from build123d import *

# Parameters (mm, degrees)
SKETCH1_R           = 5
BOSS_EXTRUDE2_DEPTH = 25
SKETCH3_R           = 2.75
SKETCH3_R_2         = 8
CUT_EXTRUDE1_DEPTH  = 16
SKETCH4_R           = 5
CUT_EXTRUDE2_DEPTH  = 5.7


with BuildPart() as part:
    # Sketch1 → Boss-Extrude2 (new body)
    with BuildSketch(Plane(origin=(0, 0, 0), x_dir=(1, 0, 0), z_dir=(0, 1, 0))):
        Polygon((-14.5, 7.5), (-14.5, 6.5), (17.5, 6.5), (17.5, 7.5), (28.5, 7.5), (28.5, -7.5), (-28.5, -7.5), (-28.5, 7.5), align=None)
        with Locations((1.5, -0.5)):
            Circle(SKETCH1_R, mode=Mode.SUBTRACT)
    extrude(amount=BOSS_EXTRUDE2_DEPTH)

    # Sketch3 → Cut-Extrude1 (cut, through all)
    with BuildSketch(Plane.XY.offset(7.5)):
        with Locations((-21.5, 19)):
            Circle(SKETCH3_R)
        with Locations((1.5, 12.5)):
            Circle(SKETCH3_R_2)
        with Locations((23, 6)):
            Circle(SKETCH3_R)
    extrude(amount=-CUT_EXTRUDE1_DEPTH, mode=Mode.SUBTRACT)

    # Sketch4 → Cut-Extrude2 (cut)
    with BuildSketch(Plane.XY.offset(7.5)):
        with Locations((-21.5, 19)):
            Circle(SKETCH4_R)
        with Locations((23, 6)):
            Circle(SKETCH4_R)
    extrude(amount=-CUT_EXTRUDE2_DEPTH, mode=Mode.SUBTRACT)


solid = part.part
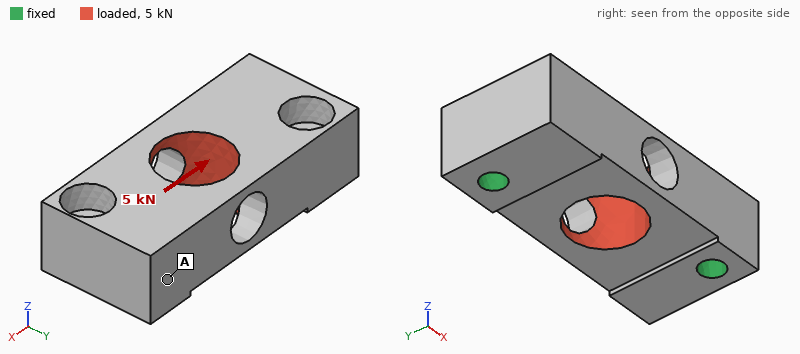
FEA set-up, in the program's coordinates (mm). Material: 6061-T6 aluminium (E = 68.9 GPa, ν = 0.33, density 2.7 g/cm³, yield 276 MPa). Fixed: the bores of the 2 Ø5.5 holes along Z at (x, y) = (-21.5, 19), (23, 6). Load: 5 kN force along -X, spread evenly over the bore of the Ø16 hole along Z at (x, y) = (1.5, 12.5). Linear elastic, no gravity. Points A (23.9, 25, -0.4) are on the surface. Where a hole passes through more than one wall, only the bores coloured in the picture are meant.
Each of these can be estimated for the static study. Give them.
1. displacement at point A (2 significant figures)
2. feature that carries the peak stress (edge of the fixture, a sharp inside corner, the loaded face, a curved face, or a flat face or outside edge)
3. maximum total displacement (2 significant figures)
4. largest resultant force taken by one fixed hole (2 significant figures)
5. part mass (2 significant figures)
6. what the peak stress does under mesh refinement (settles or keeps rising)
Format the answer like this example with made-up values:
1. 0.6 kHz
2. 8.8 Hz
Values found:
1. 8.7 µm
2. edge of the fixture
3. 10 µm
4. 2.5 kN
5. 42 g
6. keeps rising
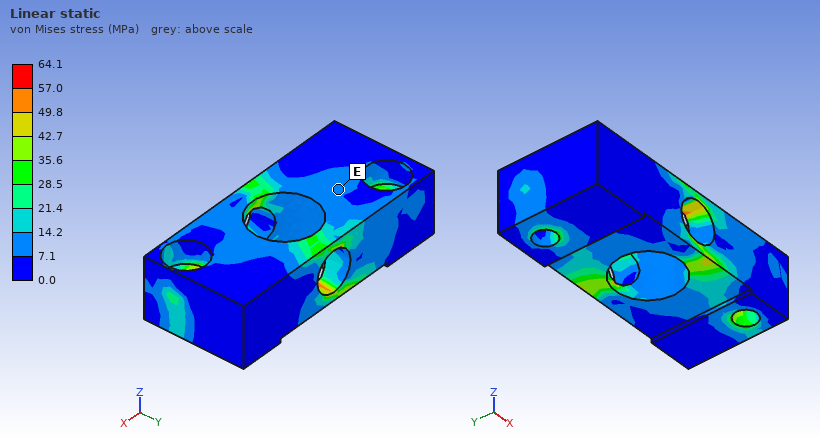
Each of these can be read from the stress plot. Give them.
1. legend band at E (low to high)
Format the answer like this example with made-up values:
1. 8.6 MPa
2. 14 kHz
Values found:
1. 7.1 to 14.2 MPa
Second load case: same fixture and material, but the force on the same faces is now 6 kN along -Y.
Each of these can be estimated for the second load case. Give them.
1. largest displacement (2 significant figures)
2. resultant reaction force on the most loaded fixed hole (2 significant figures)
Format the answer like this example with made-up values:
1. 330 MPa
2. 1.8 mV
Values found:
1. 31 µm
2. 3.1 kN
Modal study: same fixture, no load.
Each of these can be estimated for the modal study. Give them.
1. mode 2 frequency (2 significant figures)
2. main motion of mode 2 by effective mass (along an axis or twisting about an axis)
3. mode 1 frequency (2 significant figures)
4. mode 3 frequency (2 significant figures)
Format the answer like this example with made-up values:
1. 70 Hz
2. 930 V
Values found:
1. 15 kHz
2. along Z
3. 14 kHz
4. 18 kHz
